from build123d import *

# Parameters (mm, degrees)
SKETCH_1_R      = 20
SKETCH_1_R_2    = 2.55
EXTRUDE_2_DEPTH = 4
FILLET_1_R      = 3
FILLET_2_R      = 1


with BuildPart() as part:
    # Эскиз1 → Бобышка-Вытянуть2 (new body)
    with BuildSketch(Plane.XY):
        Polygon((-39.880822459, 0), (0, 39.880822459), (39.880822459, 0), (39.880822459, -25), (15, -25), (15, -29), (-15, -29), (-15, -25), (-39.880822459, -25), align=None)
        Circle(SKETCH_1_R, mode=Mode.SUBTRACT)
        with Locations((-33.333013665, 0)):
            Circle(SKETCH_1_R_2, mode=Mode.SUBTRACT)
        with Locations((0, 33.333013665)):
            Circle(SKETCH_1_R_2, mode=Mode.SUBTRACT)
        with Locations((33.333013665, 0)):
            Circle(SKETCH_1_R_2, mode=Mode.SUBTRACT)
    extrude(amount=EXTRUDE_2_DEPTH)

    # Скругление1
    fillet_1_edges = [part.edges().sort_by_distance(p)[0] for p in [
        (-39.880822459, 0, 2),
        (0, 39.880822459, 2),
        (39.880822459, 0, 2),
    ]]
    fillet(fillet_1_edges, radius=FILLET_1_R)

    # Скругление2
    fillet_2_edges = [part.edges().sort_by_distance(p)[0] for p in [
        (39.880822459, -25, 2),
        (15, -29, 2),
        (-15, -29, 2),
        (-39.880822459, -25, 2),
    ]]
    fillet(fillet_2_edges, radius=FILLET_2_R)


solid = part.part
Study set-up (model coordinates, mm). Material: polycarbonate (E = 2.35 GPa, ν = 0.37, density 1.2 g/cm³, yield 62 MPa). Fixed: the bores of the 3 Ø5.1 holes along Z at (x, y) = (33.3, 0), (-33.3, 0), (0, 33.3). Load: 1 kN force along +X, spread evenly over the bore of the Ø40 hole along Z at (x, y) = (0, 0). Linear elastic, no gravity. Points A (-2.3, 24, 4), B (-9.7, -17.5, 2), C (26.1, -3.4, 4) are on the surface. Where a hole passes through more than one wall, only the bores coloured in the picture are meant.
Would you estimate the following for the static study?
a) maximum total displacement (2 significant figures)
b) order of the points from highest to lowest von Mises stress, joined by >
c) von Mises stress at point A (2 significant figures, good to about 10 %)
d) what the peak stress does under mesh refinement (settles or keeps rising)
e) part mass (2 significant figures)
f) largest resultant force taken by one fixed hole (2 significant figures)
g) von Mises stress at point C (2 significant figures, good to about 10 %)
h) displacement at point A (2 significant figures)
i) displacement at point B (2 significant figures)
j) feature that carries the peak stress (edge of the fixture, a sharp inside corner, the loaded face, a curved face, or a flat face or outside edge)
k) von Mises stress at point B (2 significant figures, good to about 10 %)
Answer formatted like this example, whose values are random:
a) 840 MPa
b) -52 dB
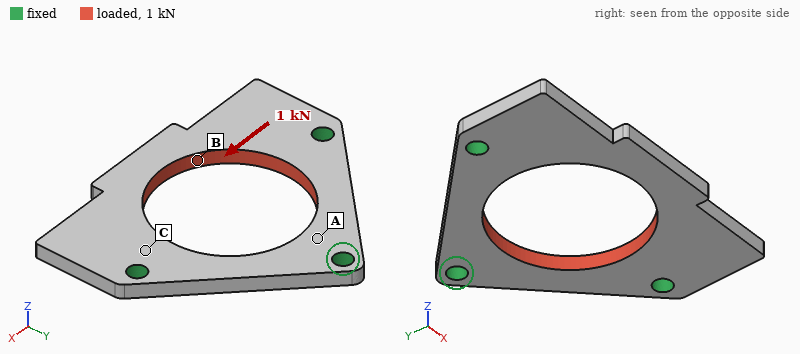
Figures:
a) 0.15 mm
b) B > C > A
c) 2.7 MPa
d) keeps rising
e) 11 g
f) 400 N
g) 7.1 MPa
h) 0.057 mm
i) 0.14 mm
j) edge of the fixture
k) 11 MPa
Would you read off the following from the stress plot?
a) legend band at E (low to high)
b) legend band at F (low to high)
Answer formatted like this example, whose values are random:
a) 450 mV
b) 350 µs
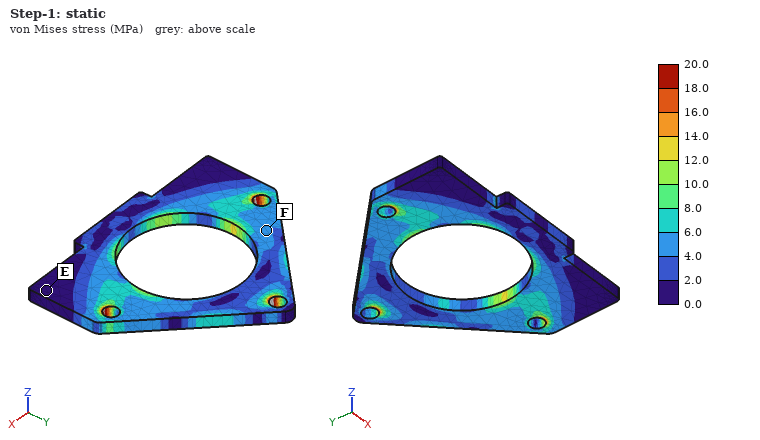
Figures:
a) 0.0 to 2.0 MPa
b) 4.0 to 6.0 MPa
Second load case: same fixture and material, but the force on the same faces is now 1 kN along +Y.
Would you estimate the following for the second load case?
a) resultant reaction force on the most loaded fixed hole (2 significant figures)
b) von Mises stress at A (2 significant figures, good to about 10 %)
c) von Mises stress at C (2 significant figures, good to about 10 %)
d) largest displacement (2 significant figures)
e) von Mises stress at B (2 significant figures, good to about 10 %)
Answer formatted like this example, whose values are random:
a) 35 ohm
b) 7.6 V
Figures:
a) 390 N
b) 4.9 MPa
c) 7.4 MPa
d) 0.16 mm
e) 5.1 MPa
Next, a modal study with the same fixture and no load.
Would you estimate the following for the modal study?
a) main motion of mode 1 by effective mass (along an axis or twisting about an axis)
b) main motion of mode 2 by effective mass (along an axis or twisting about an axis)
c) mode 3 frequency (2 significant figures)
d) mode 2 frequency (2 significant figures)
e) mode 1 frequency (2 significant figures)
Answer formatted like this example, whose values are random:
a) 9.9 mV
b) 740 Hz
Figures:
a) along Z
b) twisting about Y
c) 2200 Hz
d) 1600 Hz
e) 800 Hz
